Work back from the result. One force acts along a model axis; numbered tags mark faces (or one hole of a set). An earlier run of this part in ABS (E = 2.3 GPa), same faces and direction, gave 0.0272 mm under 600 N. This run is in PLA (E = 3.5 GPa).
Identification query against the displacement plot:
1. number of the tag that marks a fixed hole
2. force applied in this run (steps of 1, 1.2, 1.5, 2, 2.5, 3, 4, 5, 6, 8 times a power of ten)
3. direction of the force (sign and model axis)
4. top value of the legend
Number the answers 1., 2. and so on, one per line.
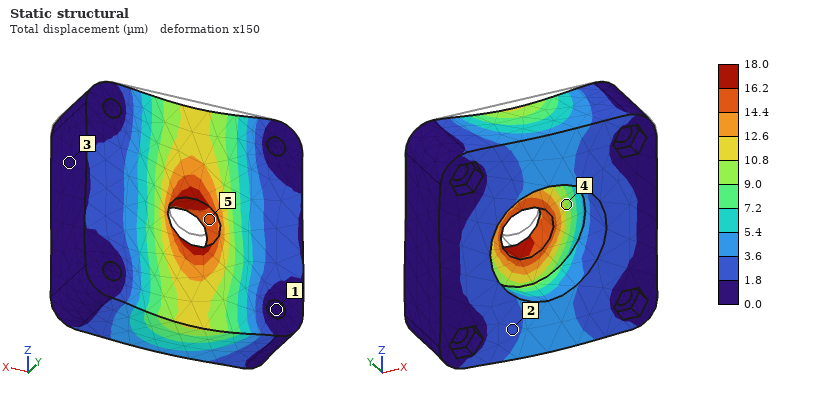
1. 1
2. 600 N
3. -Z
4. 18.0 µm
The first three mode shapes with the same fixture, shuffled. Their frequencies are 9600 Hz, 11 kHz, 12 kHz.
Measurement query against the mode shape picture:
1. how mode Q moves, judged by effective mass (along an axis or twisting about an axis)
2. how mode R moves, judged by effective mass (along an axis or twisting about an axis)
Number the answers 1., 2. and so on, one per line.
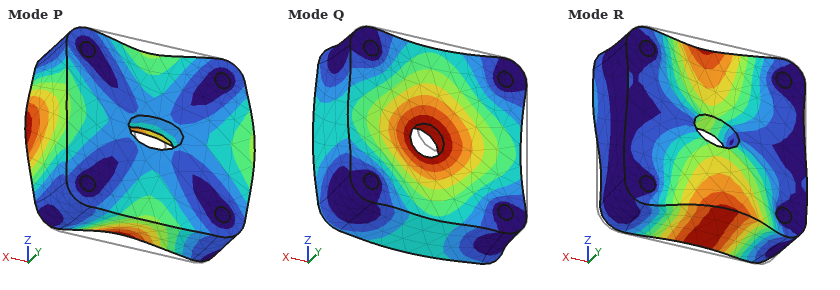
1. along Y
2. twisting about X
